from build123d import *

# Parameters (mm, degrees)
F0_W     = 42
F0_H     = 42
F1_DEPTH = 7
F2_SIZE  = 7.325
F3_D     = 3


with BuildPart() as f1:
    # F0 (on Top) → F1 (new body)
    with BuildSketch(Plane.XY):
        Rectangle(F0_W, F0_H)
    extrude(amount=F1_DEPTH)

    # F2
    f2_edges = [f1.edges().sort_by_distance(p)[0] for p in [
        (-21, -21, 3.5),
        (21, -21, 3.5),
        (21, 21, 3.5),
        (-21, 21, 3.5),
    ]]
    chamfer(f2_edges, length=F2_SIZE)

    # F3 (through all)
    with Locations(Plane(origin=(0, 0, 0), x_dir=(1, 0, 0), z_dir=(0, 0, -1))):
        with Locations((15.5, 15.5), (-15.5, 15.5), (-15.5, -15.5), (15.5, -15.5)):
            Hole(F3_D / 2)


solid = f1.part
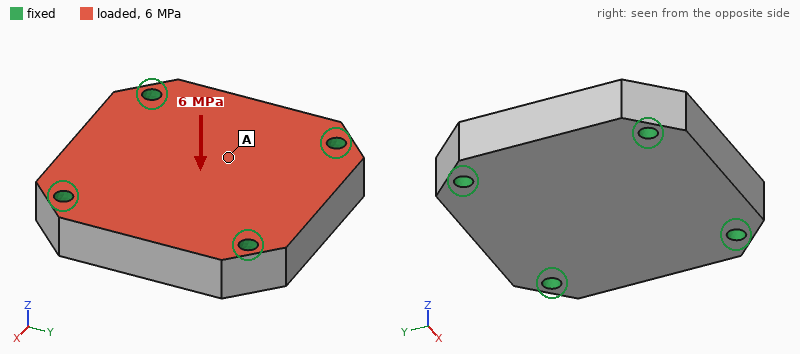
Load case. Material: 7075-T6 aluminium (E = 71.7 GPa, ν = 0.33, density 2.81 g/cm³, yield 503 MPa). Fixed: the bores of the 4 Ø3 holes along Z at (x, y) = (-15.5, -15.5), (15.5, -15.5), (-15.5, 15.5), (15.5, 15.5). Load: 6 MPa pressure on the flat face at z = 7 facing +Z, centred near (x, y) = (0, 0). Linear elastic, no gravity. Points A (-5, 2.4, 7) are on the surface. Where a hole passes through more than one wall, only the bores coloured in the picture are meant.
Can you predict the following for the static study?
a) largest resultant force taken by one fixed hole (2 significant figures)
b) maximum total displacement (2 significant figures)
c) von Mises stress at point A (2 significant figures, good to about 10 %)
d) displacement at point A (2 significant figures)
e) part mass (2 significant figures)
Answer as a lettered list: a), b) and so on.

a) 2.4 kN
b) 26 µm
c) 30 MPa
d) 24 µm
e) 32 g
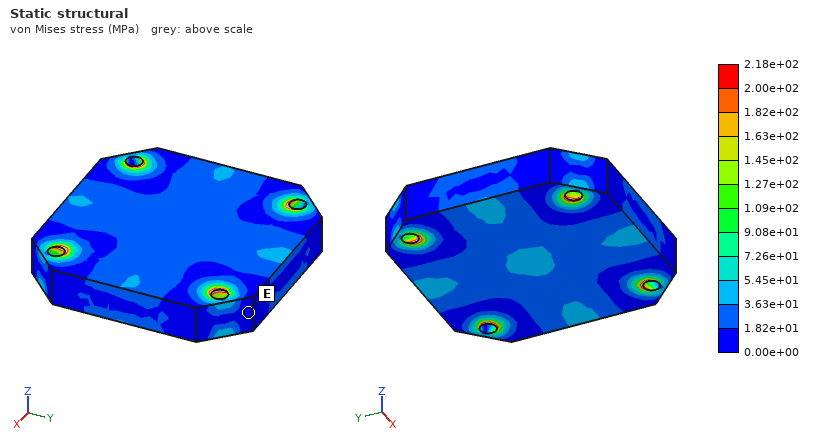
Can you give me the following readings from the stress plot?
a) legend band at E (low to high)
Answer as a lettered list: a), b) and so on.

a) 0.00e+00 to 1.82e+01 MPa
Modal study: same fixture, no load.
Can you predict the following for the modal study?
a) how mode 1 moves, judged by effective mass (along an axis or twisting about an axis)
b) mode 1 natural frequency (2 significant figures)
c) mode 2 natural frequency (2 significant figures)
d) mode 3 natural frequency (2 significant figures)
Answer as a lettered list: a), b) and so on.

a) along Z
b) 20 kHz
c) 30 kHz
d) 30 kHz
